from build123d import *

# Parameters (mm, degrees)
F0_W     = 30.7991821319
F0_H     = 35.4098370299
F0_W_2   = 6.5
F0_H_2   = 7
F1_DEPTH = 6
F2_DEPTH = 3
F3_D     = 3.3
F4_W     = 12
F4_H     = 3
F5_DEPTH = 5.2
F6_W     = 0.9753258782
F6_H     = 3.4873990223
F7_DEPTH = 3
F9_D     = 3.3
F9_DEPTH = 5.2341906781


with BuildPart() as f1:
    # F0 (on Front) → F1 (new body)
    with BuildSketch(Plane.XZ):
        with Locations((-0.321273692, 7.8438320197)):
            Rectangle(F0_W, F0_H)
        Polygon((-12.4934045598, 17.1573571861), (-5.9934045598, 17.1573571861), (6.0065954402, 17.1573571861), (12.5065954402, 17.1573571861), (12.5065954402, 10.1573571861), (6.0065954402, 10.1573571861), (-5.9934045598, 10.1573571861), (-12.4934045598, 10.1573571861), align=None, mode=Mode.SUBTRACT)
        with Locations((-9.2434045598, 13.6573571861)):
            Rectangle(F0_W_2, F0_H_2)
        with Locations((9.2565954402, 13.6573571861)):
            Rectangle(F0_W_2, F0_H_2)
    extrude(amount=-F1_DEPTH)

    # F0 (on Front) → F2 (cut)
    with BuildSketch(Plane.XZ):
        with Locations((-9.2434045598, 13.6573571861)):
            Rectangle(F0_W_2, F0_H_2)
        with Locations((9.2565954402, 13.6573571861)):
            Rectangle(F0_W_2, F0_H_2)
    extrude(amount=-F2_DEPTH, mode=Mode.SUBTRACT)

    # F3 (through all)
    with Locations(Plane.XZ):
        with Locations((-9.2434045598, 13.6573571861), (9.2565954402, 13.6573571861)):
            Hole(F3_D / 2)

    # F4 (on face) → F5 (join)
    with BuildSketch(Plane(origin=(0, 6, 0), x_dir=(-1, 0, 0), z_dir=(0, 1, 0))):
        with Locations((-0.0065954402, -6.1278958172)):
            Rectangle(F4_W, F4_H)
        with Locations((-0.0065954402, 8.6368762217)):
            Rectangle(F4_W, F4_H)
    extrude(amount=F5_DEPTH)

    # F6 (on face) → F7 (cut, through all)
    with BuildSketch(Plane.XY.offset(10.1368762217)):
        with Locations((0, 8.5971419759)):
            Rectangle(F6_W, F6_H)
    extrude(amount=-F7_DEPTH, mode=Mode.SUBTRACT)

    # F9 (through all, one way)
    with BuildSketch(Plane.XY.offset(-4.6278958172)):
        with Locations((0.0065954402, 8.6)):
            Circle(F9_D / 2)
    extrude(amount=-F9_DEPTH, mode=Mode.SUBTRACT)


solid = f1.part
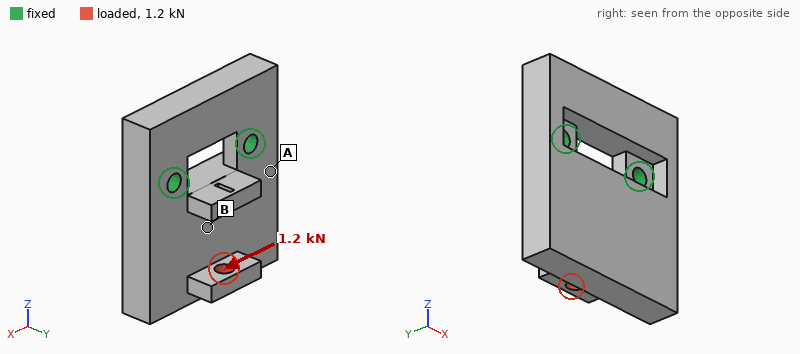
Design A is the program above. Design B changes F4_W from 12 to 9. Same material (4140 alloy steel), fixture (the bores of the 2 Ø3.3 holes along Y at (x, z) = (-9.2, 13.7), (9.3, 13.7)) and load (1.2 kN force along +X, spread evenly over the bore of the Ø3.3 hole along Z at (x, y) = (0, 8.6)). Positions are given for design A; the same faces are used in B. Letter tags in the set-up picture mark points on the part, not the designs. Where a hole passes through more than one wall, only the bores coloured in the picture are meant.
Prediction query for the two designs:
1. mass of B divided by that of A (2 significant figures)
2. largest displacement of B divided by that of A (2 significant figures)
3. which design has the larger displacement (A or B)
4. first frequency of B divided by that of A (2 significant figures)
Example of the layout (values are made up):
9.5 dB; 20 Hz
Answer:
0.98; 1.2; B; 1.0
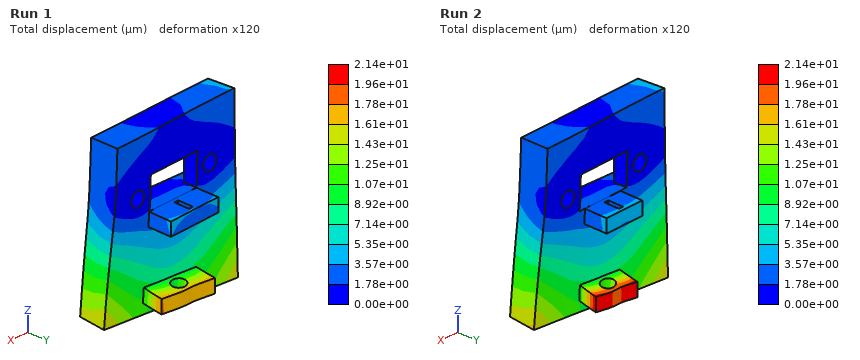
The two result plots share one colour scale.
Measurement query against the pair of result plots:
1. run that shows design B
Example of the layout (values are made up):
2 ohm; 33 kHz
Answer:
Run 2
